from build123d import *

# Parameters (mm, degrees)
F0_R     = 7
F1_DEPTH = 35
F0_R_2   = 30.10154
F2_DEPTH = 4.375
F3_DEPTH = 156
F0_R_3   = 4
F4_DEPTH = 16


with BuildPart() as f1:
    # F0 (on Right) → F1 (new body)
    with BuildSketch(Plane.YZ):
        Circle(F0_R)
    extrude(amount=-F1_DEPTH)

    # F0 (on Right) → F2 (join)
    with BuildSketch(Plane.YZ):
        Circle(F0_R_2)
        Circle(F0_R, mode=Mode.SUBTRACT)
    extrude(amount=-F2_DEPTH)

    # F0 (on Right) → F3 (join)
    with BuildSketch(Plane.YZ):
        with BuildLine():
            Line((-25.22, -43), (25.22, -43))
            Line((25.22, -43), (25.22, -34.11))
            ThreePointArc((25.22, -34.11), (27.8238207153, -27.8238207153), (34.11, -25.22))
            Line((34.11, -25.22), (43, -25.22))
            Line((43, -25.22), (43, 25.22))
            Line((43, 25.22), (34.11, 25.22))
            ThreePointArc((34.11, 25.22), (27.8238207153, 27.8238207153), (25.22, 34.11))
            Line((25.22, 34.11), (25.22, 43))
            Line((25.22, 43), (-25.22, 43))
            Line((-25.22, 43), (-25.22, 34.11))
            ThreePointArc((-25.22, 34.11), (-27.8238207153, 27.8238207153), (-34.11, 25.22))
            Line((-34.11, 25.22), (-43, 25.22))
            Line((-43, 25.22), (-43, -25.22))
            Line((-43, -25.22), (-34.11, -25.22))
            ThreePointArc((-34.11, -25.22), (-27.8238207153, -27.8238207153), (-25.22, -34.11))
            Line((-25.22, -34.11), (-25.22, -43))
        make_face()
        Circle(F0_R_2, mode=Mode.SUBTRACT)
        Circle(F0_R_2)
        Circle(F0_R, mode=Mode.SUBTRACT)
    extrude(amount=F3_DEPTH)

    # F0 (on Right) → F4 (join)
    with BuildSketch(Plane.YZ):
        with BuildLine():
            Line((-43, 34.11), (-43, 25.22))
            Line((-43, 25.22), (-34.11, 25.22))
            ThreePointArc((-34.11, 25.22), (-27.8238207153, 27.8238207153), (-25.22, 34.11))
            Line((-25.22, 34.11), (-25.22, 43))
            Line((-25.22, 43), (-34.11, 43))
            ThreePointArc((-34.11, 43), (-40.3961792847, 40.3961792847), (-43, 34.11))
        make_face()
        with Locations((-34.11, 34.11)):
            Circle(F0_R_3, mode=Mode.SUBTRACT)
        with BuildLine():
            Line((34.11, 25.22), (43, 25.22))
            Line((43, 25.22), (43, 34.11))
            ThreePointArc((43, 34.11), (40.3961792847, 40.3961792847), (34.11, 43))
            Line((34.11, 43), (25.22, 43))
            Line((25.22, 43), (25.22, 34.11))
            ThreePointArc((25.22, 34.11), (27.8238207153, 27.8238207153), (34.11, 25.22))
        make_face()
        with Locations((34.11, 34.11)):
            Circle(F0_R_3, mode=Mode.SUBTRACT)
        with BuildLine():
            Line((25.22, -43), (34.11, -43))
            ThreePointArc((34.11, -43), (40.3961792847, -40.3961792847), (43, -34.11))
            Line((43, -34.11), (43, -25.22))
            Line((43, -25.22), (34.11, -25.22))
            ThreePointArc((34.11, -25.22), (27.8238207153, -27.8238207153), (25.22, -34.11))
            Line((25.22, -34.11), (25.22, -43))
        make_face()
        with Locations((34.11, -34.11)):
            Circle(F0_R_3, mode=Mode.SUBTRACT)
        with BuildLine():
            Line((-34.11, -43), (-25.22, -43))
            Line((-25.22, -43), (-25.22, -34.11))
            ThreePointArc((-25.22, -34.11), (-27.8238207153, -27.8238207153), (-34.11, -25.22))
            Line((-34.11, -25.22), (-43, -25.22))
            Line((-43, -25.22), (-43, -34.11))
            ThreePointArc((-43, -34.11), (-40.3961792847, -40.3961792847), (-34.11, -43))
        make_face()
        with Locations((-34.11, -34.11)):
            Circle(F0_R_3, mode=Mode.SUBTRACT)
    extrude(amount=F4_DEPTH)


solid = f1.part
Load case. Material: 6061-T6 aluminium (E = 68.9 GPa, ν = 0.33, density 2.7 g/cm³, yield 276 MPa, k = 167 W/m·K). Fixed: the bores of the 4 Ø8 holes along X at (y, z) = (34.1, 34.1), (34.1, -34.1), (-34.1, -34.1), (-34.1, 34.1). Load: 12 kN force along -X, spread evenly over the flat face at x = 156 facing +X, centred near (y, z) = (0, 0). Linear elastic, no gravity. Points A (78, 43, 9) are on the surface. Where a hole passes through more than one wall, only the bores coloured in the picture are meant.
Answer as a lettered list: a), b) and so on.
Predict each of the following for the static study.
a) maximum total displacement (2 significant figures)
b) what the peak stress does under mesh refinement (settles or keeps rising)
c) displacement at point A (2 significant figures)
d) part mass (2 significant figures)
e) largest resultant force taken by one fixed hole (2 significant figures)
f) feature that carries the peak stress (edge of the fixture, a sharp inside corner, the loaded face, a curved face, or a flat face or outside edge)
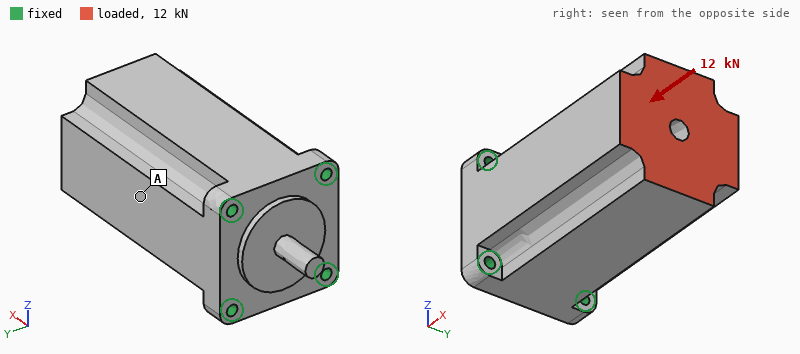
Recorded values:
a) 8.0 µm
b) keeps rising
c) 5.7 µm
d) 2.6 kg
e) 3.1 kN
f) edge of the fixture
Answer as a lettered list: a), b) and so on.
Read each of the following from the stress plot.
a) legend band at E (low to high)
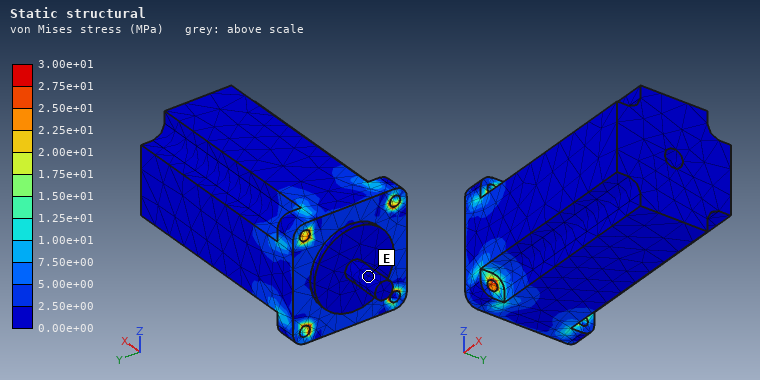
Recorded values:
a) 0.00e+00 to 2.50e+00 MPa
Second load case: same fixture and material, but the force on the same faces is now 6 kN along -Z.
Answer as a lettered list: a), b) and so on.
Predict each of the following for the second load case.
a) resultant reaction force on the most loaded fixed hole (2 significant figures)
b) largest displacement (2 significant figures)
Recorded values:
a) 7.0 kN
b) 77 µm
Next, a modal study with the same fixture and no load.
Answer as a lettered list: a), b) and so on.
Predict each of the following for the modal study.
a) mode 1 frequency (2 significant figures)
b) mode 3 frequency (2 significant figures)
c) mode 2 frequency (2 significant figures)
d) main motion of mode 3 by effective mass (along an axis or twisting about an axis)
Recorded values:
a) 1600 Hz
b) 4700 Hz
c) 1600 Hz
d) twisting about X
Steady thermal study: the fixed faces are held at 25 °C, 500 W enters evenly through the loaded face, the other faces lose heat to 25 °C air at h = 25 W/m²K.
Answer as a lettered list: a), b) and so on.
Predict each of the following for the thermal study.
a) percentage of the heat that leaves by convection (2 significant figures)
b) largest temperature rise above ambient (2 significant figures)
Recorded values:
a) 14 %
b) 83 K
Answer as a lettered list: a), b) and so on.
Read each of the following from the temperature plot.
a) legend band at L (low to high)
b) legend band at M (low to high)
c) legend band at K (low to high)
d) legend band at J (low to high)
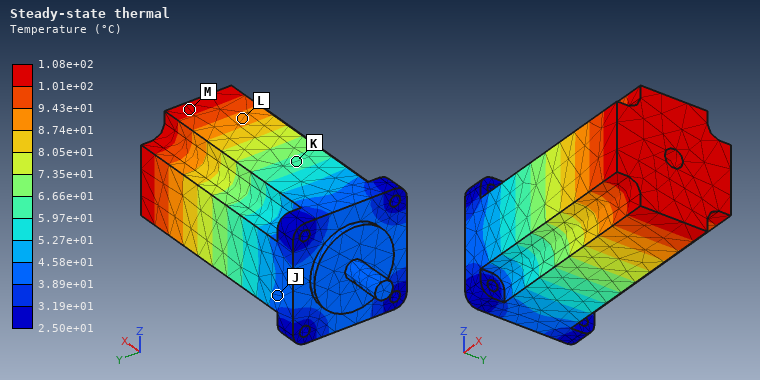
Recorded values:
a) 8.74e+01 to 9.43e+01 °C
b) 1.01e+02 to 1.08e+02 °C
c) 5.97e+01 to 6.66e+01 °C
d) 3.89e+01 to 4.58e+01 °C
